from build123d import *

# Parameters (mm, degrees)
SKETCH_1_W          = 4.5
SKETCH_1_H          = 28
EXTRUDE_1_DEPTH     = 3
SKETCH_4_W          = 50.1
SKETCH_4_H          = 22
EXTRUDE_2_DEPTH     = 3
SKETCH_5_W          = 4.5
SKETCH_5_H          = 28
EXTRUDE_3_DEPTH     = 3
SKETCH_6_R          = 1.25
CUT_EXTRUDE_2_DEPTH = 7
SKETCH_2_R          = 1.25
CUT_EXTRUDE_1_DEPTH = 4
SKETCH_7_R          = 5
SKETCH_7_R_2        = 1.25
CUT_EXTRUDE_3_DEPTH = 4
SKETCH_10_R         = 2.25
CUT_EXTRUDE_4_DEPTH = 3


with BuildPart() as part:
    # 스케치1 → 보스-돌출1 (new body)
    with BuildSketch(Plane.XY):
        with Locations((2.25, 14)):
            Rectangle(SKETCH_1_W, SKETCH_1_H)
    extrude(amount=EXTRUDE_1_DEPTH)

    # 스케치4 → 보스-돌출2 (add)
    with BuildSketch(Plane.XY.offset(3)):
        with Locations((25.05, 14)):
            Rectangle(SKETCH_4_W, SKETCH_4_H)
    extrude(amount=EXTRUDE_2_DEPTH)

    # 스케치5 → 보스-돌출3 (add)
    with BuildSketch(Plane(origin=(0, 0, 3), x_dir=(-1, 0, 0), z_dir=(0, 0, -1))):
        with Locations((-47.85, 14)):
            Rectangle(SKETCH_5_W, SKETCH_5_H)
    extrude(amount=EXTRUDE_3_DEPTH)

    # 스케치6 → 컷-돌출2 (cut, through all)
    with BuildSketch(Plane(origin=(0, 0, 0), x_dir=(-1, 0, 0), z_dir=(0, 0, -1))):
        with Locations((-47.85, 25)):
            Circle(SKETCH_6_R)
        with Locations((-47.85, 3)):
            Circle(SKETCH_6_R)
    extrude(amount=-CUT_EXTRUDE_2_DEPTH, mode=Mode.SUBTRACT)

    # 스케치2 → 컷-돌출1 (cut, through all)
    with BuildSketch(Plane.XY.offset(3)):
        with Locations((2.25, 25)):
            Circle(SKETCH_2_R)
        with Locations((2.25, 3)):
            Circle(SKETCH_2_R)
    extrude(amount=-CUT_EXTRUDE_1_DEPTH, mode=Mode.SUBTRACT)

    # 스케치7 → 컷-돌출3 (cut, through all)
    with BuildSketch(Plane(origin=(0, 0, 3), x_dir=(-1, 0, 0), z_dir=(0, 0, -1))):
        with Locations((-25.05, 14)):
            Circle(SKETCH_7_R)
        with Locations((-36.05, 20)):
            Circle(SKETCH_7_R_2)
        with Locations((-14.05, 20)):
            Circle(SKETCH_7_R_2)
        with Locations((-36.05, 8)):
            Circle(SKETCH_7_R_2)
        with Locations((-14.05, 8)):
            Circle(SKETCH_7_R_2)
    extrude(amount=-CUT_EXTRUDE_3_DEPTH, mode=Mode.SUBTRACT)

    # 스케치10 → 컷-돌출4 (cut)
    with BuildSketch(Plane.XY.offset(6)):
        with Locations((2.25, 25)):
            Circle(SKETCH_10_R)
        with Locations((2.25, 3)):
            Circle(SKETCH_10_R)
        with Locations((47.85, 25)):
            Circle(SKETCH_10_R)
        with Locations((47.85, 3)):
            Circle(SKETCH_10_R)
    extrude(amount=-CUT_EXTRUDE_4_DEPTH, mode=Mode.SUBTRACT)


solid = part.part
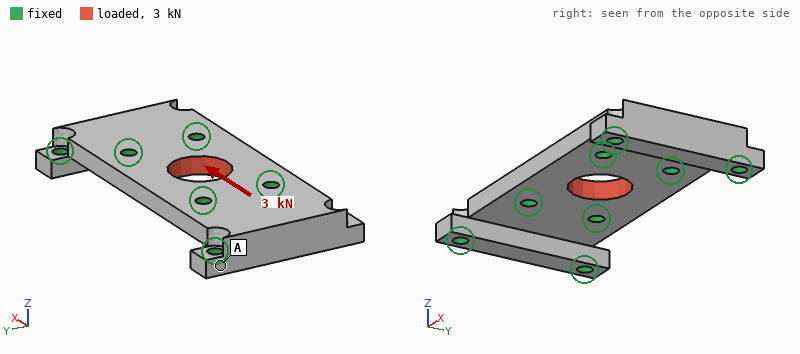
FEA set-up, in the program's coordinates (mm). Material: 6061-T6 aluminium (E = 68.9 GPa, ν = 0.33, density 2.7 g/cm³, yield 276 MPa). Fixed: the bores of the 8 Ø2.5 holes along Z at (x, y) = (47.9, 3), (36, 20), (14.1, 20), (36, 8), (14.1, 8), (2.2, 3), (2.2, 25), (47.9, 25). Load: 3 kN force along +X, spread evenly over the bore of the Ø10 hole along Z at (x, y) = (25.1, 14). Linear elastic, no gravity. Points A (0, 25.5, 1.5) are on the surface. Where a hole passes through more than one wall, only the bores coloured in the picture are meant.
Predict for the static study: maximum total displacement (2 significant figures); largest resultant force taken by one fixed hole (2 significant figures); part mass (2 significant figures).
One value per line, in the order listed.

4.6 µm
740 N
9.8 g
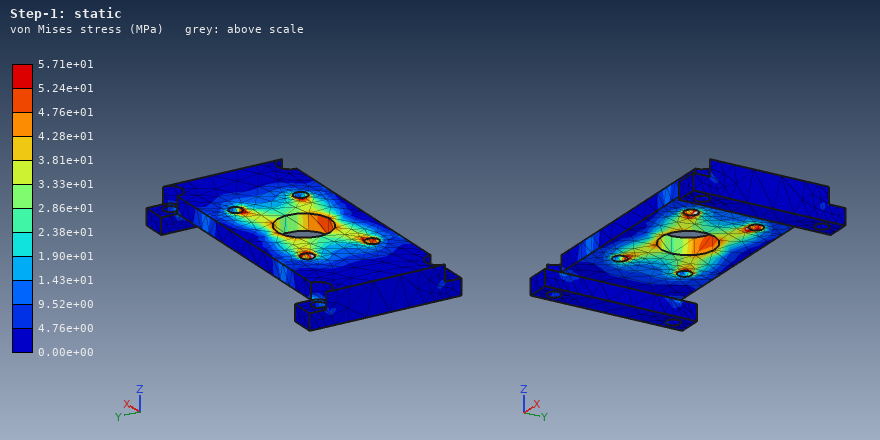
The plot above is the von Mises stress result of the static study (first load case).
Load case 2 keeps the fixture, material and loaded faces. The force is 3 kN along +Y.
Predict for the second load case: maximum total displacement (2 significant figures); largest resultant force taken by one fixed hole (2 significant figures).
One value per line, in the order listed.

12 µm
830 N
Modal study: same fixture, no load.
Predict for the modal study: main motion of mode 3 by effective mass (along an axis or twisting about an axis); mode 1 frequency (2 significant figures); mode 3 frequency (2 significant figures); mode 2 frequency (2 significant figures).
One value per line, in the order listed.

twisting about Y
31 kHz
41 kHz
33 kHz
